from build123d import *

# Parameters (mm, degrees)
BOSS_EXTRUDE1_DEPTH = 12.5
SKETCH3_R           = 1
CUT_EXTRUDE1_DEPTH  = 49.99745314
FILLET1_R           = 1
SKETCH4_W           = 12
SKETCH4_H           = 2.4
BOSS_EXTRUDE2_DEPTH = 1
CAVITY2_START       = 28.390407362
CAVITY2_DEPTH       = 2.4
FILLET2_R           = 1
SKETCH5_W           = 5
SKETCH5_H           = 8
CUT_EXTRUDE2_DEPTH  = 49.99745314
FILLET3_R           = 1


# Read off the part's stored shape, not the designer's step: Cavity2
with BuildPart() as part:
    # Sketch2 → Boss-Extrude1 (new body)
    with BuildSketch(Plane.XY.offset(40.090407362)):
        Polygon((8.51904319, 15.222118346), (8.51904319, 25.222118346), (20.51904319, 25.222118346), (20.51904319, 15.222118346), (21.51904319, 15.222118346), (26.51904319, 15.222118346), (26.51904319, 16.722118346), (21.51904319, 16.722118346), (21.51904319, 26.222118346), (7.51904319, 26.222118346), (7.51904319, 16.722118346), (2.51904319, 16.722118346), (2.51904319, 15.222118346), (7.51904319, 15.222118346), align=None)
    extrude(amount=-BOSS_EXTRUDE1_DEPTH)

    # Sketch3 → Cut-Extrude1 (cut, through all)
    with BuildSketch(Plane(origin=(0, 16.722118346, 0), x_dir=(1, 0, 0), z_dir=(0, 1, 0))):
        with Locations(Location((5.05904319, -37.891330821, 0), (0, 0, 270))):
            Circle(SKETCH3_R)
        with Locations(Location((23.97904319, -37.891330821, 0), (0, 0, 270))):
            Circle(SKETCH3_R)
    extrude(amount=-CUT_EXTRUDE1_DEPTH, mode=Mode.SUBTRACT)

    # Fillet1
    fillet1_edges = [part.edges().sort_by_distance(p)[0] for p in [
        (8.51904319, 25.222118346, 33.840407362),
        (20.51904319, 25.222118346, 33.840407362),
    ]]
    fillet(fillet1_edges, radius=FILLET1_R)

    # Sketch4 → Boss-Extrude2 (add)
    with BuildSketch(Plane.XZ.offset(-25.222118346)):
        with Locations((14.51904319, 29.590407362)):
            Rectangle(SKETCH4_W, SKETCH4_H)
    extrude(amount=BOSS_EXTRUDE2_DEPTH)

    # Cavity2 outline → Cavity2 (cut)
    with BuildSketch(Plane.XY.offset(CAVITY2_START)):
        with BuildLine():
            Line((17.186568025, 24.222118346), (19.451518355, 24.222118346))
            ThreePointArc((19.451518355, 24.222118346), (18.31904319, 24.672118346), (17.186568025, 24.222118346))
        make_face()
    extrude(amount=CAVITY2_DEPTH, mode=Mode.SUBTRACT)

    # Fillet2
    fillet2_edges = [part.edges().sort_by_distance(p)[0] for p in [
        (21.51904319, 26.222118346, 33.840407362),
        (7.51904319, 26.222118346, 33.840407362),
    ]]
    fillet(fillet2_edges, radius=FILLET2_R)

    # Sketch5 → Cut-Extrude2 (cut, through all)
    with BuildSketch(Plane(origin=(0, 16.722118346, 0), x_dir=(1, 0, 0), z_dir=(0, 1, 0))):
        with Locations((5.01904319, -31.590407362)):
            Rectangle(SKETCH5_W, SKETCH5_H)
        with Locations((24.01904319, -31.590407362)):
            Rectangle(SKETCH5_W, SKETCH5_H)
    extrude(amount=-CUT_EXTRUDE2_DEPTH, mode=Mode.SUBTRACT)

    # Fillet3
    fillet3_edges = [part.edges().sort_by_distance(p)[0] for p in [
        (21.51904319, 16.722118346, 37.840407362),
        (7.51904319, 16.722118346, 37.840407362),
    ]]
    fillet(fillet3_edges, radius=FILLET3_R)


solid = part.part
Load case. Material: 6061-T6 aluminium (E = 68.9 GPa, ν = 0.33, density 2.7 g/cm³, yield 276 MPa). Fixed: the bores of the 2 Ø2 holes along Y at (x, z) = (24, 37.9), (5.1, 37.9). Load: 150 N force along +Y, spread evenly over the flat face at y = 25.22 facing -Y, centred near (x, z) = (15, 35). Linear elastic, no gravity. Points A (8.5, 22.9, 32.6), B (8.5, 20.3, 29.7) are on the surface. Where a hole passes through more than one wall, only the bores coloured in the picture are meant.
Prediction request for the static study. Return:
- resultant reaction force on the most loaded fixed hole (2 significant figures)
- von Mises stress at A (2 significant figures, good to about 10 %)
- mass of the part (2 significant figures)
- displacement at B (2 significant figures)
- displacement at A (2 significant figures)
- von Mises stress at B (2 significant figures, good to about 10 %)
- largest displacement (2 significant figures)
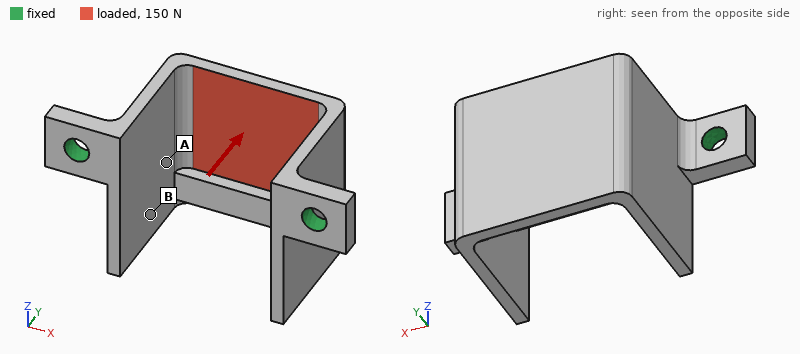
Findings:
78 N
35 MPa
1.4 g
28 µm
26 µm
13 MPa
47 µm
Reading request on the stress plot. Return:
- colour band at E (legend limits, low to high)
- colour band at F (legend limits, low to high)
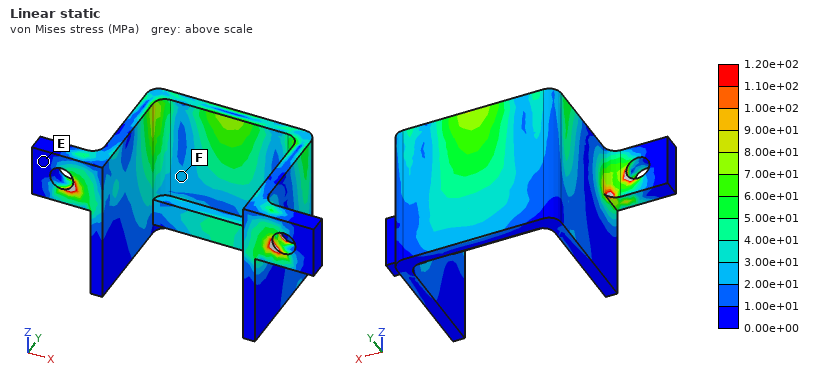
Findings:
0.00e+00 to 1.00e+01 MPa
2.00e+01 to 3.00e+01 MPa
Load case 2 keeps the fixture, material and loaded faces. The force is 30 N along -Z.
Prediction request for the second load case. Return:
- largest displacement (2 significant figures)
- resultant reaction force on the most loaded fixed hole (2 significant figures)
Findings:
32 µm
15 N
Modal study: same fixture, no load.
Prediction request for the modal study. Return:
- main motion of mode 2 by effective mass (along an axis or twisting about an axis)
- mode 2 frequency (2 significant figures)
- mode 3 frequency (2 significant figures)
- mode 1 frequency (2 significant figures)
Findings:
along X
5900 Hz
8600 Hz
5400 Hz
